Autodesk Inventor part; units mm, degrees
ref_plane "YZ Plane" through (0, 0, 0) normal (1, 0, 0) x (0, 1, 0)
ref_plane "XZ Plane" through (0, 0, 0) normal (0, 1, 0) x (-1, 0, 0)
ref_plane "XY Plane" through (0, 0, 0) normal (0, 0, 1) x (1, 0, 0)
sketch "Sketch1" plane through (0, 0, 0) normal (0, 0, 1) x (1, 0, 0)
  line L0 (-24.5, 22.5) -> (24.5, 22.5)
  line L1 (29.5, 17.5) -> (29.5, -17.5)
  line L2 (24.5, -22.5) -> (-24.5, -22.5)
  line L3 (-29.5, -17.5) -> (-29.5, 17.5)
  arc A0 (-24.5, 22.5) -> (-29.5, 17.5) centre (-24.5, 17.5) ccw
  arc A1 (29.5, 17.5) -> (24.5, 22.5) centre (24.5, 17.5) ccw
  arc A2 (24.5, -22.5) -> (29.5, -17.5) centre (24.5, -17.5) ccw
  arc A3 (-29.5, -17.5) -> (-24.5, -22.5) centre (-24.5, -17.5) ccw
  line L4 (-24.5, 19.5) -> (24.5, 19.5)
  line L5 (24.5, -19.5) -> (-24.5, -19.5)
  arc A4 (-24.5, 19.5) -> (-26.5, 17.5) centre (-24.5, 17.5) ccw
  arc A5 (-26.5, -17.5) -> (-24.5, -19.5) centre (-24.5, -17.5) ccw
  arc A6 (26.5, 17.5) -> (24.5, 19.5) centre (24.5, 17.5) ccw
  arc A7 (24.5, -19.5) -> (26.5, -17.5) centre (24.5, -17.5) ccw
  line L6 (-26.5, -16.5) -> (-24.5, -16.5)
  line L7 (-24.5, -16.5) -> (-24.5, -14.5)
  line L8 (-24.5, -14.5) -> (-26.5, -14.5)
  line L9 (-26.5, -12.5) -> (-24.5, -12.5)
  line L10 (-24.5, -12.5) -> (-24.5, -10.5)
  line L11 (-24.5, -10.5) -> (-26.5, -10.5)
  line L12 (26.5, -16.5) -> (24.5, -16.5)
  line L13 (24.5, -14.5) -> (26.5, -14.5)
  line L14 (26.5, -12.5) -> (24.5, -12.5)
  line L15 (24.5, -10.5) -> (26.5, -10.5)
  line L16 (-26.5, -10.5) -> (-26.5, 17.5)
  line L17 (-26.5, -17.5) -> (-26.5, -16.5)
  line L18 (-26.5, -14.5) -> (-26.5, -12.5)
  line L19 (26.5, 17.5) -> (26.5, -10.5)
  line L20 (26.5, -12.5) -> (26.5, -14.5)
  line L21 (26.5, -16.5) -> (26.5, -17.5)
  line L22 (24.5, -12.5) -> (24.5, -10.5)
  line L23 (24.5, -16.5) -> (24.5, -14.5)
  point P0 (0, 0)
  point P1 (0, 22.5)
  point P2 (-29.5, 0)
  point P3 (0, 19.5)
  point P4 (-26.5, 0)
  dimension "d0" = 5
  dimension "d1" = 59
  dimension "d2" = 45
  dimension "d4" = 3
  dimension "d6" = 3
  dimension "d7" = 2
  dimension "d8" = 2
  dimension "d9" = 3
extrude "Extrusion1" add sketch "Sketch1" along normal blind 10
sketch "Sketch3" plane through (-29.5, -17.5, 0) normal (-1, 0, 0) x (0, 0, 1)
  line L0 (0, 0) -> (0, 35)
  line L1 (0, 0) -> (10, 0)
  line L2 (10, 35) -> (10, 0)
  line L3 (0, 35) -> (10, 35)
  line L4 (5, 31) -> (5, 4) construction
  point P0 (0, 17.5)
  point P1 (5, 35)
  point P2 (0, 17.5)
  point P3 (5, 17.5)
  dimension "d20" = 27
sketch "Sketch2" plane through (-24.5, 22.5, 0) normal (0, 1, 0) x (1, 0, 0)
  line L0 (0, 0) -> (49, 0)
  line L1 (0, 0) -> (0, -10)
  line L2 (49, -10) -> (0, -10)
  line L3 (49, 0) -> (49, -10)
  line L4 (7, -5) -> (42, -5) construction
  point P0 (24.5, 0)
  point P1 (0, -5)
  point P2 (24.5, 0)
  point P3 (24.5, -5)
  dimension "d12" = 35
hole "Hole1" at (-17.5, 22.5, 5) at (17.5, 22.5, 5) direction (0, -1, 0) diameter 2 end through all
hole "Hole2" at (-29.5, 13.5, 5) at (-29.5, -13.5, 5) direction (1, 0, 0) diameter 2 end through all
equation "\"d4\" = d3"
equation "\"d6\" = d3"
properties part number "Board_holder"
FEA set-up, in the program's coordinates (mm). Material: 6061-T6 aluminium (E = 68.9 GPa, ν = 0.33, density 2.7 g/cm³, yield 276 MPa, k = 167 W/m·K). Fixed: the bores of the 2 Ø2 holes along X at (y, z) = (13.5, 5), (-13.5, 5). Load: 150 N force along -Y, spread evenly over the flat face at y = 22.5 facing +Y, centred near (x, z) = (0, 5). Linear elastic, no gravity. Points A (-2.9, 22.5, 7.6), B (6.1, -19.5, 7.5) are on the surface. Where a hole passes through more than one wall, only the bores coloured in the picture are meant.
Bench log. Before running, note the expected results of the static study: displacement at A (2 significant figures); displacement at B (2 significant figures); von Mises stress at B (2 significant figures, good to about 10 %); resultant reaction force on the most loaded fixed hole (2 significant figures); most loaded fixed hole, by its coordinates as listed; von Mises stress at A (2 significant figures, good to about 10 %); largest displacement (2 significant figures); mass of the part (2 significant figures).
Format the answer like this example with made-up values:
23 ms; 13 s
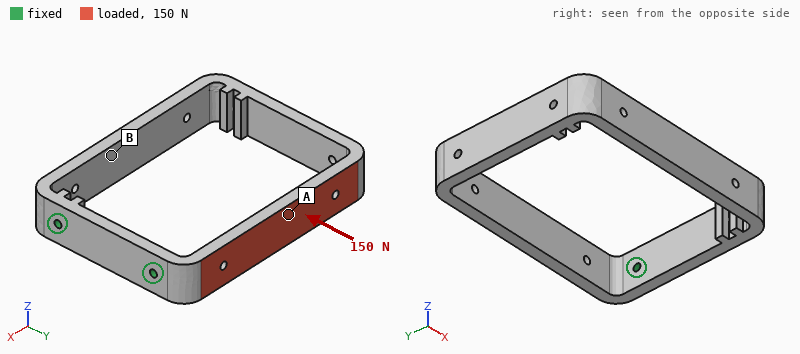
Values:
0.45 mm; 0.22 mm; 17 MPa; 120 N; (13.5, 5); 43 MPa; 0.64 mm; 16 g
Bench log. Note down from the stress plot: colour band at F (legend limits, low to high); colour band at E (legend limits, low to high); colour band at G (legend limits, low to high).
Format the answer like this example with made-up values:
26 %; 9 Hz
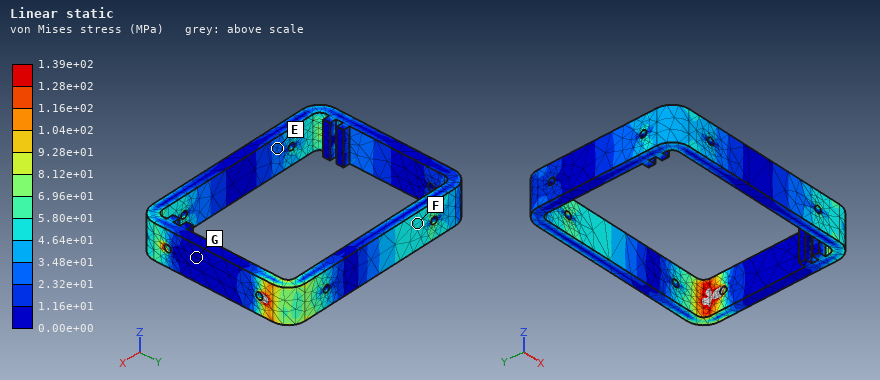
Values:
4.64e+01 to 5.80e+01 MPa; 2.32e+01 to 3.48e+01 MPa; 0.00e+00 to 1.16e+01 MPa
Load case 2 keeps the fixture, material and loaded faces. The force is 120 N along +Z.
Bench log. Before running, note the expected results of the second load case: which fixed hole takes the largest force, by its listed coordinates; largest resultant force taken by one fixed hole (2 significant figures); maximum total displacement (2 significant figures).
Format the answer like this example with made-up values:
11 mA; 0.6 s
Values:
(13.5, 5); 150 N; 0.51 mm
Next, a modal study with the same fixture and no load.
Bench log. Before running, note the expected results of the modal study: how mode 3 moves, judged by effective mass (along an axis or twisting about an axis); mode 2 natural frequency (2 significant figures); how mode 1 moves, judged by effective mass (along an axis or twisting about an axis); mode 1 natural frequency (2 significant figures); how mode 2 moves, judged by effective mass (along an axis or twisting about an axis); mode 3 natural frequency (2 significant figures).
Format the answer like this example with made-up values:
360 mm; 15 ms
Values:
twisting about X; 810 Hz; along Y; 680 Hz; along Z; 1600 Hz
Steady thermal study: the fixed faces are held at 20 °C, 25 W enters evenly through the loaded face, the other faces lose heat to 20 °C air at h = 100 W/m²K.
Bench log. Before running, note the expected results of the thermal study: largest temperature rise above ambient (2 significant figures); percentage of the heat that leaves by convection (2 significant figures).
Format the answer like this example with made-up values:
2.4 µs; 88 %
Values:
70 K; 43 %
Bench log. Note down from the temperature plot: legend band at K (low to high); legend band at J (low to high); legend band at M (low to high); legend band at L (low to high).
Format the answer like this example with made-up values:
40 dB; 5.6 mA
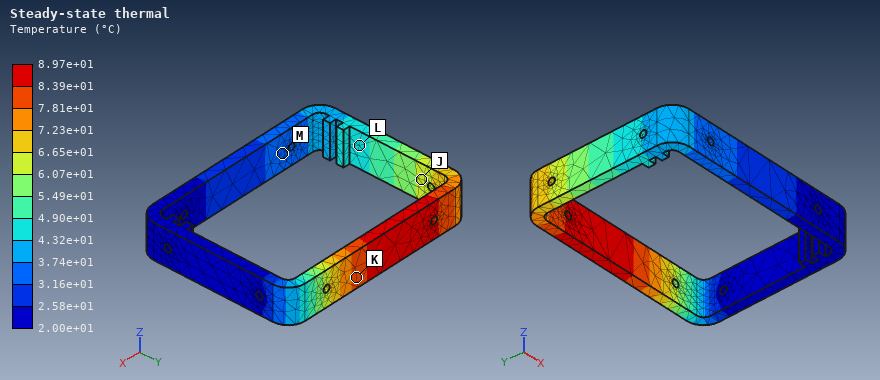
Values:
7.81e+01 to 8.39e+01 °C; 6.07e+01 to 6.65e+01 °C; 3.16e+01 to 3.74e+01 °C; 4.32e+01 to 4.90e+01 °C
